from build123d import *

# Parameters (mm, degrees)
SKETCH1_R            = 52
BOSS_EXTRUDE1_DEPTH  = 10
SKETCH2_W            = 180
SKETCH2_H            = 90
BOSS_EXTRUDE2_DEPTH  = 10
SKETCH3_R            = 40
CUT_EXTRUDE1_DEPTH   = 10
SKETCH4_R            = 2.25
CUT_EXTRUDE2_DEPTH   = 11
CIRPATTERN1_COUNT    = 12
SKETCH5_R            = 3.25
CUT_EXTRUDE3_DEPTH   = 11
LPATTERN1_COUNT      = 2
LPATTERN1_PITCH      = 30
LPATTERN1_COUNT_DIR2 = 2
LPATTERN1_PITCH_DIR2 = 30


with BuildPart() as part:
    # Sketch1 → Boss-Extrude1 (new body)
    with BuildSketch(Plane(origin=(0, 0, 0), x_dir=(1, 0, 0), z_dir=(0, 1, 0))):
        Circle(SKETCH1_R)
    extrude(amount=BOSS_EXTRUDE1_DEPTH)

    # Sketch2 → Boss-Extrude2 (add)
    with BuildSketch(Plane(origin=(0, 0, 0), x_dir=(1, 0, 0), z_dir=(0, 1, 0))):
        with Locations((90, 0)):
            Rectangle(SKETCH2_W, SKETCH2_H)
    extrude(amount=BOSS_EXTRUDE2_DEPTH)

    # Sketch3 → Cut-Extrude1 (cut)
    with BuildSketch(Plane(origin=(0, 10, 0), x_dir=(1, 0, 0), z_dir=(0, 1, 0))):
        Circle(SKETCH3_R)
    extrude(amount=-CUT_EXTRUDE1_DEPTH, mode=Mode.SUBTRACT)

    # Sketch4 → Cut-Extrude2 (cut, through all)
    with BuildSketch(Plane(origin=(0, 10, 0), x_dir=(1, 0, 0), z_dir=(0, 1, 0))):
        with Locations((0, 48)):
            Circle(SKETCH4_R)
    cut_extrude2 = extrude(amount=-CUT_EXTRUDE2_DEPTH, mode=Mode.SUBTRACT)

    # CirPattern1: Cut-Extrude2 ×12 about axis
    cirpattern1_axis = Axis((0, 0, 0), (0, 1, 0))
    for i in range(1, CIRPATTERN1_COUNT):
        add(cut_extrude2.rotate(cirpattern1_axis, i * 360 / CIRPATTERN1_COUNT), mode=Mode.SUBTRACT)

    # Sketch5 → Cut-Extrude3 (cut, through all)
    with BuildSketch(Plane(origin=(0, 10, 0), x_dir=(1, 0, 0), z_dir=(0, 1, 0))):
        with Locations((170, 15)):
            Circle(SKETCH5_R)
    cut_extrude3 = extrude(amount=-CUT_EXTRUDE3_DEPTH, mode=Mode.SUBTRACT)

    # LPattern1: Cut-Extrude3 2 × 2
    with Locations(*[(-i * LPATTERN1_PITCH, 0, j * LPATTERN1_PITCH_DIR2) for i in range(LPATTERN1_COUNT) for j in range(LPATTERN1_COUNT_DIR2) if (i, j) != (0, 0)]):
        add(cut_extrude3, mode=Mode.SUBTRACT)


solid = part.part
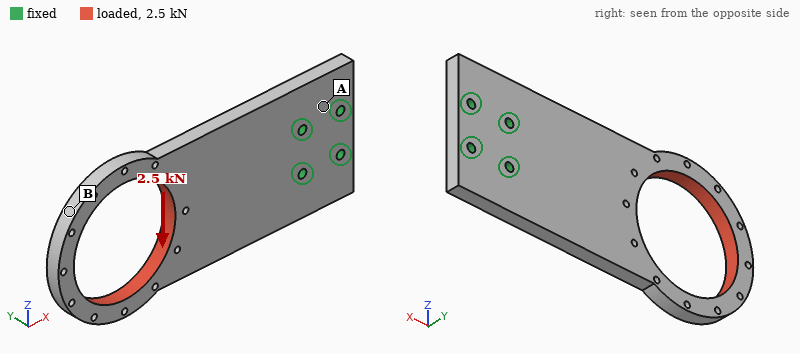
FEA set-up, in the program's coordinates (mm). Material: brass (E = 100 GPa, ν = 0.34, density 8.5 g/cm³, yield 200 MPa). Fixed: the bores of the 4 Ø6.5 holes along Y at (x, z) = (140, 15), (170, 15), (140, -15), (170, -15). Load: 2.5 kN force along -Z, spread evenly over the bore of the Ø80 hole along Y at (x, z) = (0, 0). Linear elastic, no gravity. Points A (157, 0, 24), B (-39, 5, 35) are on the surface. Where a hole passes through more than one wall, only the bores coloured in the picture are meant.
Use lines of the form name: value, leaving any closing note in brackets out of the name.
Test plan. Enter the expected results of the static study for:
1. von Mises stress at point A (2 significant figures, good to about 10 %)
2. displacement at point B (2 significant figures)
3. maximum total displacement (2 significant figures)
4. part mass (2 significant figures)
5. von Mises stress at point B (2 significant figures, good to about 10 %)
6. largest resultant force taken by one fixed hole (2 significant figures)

von Mises stress at point A: 16 MPa
displacement at point B: 0.27 mm
maximum total displacement: 0.27 mm
part mass: 1.3 kg
von Mises stress at point B: 36 MPa
largest resultant force taken by one fixed hole: 5.9 kN
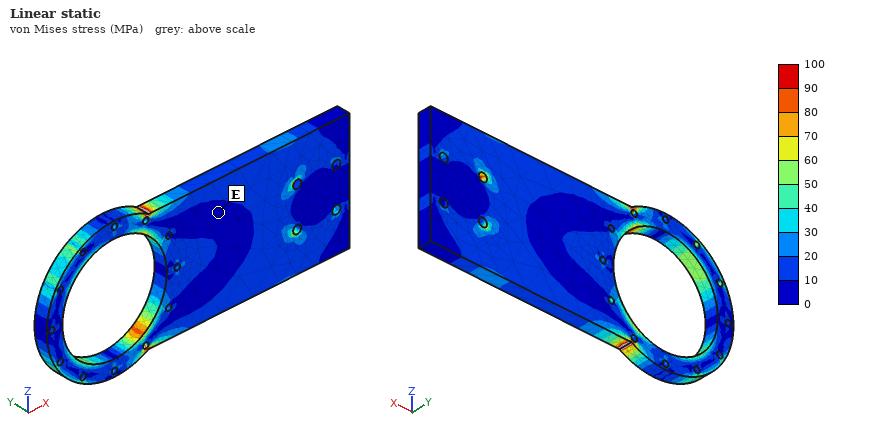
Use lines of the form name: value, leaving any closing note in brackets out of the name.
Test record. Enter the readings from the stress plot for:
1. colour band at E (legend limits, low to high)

colour band at E: 0 to 10 MPa
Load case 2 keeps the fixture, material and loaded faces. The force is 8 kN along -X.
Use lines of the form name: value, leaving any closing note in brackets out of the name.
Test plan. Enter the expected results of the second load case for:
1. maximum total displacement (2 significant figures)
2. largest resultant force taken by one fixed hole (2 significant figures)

maximum total displacement: 0.10 mm
largest resultant force taken by one fixed hole: 3.2 kN
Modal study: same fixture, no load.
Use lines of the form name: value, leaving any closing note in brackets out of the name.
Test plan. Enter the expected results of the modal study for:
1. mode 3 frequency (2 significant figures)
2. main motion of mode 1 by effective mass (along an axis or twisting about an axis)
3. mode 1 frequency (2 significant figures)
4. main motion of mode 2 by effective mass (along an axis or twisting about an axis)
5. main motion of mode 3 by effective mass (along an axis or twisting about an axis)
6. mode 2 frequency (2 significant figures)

mode 3 frequency: 780 Hz
main motion of mode 1 by effective mass: along Y
mode 1 frequency: 220 Hz
main motion of mode 2 by effective mass: twisting about X
main motion of mode 3 by effective mass: along Y
mode 2 frequency: 650 Hz
